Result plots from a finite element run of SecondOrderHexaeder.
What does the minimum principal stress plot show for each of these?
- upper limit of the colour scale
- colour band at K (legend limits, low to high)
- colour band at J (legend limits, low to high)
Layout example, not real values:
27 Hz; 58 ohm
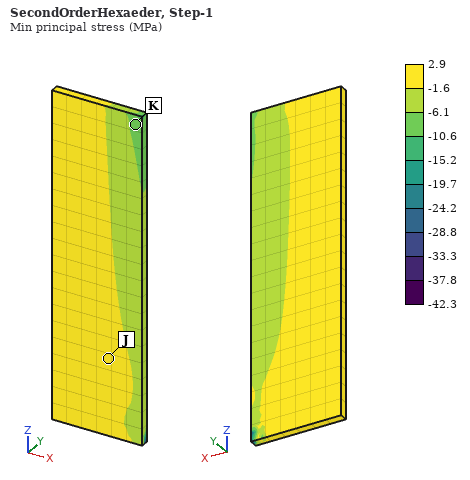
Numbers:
2.9 MPa; -10.6 to -6.1 MPa; -1.6 to 2.9 MPa
